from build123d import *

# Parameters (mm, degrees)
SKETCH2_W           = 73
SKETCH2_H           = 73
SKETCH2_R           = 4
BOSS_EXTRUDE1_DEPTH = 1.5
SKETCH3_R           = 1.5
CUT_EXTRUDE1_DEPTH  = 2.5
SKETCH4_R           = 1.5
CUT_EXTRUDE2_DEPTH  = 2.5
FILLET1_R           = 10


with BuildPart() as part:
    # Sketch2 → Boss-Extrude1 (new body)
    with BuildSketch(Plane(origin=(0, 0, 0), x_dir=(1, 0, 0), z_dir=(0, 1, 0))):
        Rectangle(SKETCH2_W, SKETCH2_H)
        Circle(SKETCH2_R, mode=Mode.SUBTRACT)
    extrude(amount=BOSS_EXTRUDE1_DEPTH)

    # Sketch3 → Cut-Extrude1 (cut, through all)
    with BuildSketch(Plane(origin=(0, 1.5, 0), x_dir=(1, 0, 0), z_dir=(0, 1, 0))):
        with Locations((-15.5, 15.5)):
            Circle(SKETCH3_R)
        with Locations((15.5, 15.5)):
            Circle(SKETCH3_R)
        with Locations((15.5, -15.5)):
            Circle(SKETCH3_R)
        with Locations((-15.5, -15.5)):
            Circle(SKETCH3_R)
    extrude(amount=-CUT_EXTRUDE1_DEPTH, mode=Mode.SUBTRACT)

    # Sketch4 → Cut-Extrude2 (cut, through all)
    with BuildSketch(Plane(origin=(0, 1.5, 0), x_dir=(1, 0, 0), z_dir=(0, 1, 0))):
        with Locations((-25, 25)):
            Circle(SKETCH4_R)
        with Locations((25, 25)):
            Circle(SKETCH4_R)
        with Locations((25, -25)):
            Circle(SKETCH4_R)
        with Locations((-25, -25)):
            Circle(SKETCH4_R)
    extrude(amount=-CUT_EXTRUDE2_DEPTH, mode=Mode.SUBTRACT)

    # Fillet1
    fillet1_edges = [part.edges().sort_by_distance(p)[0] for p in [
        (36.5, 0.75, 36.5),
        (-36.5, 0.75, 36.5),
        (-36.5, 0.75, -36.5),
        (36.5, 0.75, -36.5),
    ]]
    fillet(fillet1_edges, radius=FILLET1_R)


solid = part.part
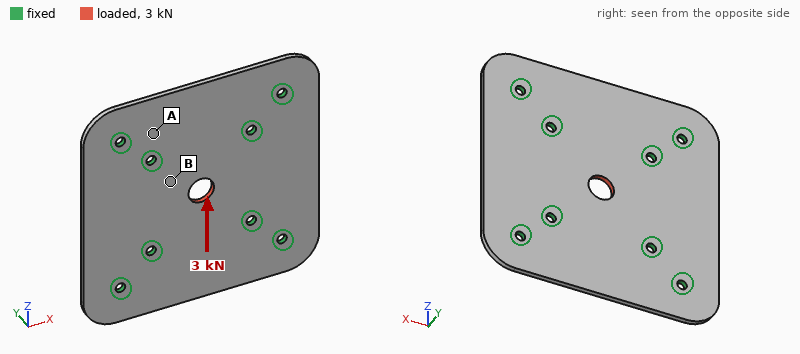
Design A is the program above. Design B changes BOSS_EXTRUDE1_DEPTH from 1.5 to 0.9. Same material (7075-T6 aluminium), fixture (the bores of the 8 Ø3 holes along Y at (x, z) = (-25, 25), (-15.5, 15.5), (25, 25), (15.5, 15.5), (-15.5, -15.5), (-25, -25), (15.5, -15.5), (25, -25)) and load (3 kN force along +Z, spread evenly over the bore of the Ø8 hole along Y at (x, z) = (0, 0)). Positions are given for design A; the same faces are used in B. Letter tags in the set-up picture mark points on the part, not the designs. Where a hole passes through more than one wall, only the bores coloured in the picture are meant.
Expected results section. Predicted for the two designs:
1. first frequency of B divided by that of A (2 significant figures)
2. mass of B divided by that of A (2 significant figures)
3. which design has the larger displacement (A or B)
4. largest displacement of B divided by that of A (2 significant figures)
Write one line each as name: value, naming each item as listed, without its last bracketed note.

first frequency of B divided by that of A: 0.62
mass of B divided by that of A: 0.60
which design has the larger displacement: B
largest displacement of B divided by that of A: 1.7
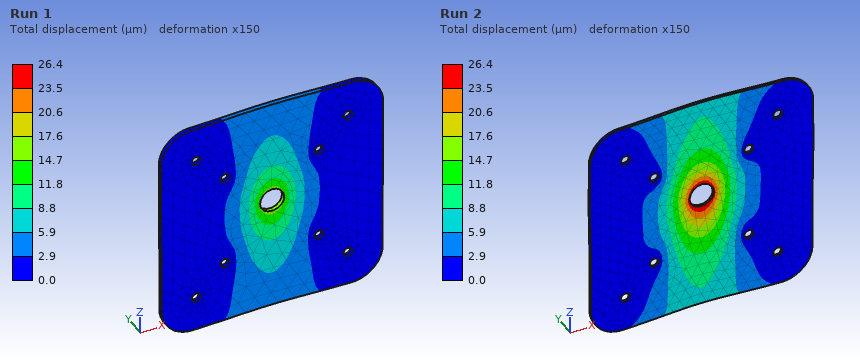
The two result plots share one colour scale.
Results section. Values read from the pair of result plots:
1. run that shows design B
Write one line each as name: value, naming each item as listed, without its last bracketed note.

run that shows design B: Run 2
